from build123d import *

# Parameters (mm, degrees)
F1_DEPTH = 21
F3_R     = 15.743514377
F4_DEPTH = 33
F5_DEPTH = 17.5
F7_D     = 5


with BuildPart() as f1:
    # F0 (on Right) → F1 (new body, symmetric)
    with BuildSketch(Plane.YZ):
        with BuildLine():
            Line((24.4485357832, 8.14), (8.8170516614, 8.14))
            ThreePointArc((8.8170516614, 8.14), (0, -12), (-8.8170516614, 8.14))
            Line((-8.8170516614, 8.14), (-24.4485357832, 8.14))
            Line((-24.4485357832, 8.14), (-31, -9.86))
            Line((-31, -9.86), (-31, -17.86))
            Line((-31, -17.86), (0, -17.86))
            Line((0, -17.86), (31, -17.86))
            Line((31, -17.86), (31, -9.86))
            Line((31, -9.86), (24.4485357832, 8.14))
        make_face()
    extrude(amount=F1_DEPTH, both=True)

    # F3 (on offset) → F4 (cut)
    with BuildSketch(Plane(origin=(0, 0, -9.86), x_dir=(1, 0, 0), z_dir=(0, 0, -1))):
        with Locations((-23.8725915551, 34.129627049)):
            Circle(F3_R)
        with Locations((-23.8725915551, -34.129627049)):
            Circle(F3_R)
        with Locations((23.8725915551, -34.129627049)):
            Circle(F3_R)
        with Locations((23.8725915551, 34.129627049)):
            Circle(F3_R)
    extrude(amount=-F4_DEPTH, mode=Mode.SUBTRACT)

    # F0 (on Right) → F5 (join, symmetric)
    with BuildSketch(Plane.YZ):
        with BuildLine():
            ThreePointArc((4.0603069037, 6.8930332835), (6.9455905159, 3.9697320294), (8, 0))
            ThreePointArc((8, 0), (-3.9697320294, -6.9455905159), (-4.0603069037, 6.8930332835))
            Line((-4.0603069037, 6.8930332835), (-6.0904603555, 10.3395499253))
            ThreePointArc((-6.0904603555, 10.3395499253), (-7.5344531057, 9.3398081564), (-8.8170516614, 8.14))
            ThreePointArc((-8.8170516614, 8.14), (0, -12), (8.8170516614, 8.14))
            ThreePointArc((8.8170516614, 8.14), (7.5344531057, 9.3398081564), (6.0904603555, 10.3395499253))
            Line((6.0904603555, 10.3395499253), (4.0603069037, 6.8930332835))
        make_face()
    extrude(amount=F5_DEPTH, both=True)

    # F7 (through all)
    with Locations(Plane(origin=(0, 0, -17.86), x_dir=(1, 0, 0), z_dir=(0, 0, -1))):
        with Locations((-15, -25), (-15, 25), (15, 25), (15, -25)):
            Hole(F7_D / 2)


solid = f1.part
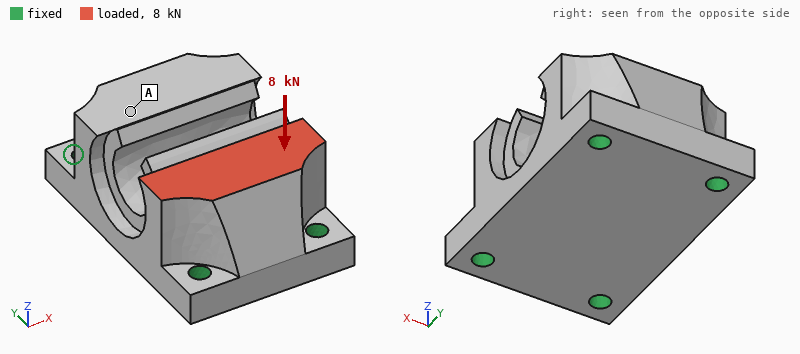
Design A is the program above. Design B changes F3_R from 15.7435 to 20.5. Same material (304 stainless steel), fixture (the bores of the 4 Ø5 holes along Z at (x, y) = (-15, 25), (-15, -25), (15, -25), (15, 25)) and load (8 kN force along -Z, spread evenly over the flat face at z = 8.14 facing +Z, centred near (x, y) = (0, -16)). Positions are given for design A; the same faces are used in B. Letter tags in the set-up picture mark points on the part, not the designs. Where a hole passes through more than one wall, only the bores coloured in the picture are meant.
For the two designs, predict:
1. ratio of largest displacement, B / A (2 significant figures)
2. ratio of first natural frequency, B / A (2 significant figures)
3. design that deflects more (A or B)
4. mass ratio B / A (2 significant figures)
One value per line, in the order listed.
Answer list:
1.2
1.0
B
0.86
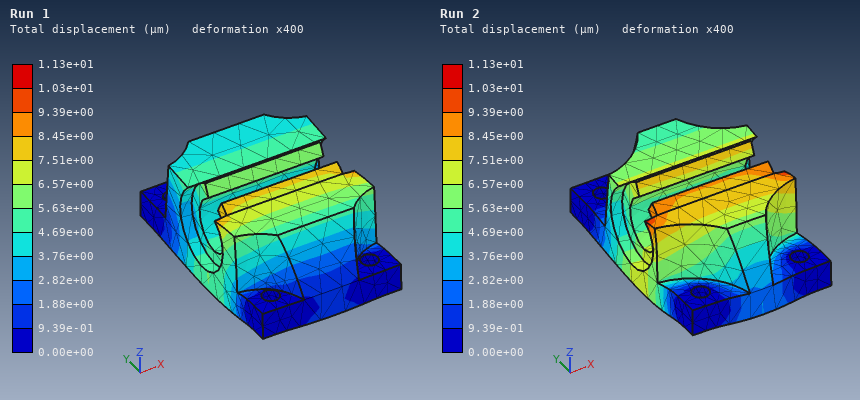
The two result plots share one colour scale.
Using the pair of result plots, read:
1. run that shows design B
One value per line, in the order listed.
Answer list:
Run 2
